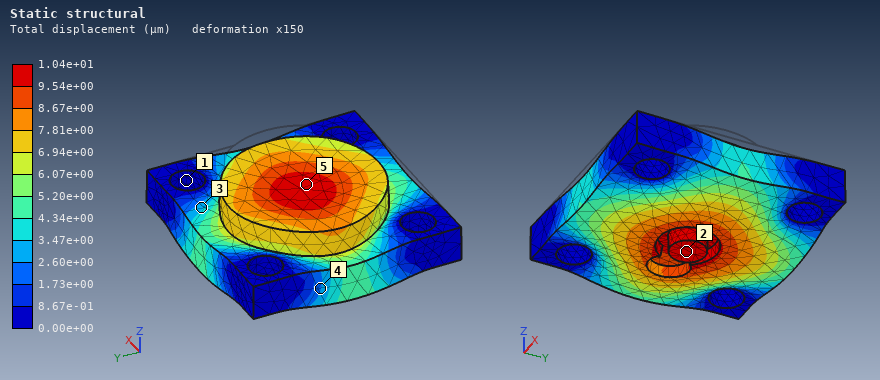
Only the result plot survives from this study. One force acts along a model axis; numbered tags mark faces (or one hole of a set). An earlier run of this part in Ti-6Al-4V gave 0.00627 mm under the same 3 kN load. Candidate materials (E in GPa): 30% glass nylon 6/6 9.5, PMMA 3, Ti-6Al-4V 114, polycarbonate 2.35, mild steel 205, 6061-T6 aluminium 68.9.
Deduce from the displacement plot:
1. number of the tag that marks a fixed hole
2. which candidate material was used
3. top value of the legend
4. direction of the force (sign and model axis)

1
6061-T6 aluminium
1.04e+01 µm
-Z
